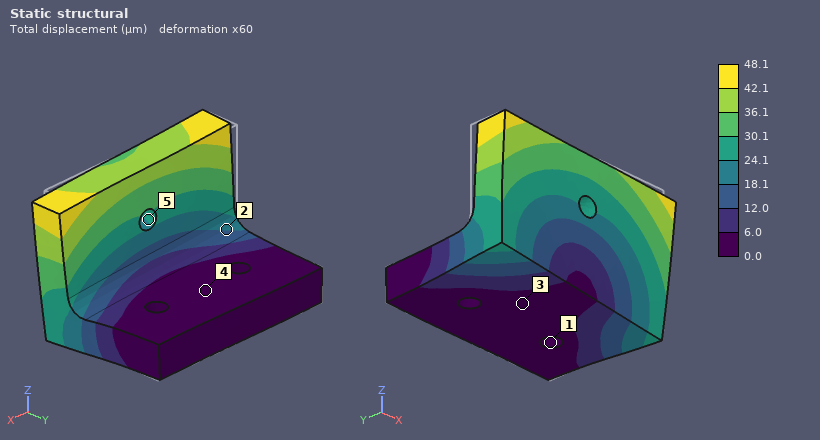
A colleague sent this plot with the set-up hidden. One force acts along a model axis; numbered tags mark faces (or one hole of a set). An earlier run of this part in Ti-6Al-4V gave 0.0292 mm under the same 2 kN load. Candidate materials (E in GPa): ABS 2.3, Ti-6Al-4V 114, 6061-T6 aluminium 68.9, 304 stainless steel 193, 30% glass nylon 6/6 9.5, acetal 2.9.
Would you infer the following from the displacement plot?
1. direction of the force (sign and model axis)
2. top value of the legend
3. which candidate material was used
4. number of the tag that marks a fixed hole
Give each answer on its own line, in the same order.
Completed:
+X
48.1 µm
6061-T6 aluminium
1
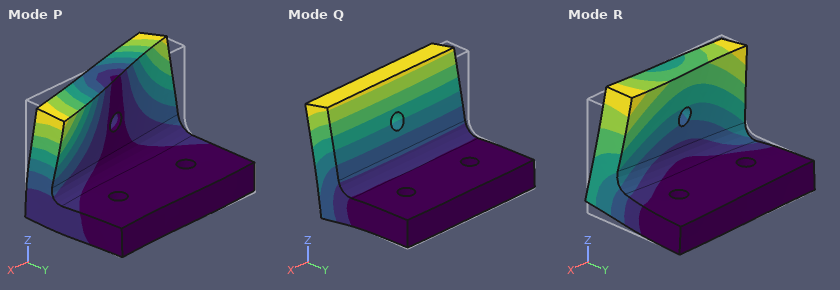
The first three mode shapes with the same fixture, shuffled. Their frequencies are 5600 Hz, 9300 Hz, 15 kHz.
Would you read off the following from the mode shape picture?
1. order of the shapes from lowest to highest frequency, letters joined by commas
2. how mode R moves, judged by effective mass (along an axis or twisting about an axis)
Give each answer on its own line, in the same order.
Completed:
Q, R, P
along X
